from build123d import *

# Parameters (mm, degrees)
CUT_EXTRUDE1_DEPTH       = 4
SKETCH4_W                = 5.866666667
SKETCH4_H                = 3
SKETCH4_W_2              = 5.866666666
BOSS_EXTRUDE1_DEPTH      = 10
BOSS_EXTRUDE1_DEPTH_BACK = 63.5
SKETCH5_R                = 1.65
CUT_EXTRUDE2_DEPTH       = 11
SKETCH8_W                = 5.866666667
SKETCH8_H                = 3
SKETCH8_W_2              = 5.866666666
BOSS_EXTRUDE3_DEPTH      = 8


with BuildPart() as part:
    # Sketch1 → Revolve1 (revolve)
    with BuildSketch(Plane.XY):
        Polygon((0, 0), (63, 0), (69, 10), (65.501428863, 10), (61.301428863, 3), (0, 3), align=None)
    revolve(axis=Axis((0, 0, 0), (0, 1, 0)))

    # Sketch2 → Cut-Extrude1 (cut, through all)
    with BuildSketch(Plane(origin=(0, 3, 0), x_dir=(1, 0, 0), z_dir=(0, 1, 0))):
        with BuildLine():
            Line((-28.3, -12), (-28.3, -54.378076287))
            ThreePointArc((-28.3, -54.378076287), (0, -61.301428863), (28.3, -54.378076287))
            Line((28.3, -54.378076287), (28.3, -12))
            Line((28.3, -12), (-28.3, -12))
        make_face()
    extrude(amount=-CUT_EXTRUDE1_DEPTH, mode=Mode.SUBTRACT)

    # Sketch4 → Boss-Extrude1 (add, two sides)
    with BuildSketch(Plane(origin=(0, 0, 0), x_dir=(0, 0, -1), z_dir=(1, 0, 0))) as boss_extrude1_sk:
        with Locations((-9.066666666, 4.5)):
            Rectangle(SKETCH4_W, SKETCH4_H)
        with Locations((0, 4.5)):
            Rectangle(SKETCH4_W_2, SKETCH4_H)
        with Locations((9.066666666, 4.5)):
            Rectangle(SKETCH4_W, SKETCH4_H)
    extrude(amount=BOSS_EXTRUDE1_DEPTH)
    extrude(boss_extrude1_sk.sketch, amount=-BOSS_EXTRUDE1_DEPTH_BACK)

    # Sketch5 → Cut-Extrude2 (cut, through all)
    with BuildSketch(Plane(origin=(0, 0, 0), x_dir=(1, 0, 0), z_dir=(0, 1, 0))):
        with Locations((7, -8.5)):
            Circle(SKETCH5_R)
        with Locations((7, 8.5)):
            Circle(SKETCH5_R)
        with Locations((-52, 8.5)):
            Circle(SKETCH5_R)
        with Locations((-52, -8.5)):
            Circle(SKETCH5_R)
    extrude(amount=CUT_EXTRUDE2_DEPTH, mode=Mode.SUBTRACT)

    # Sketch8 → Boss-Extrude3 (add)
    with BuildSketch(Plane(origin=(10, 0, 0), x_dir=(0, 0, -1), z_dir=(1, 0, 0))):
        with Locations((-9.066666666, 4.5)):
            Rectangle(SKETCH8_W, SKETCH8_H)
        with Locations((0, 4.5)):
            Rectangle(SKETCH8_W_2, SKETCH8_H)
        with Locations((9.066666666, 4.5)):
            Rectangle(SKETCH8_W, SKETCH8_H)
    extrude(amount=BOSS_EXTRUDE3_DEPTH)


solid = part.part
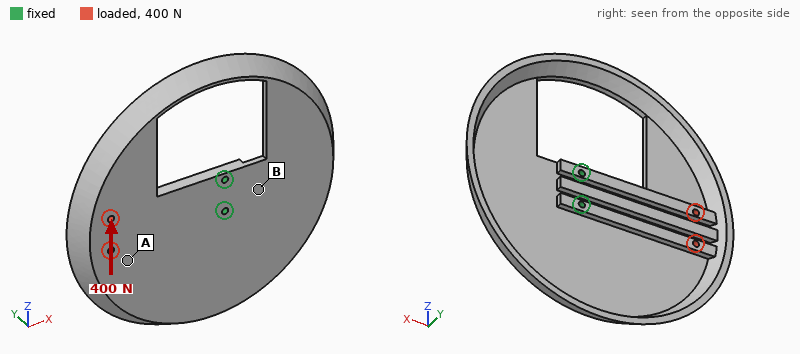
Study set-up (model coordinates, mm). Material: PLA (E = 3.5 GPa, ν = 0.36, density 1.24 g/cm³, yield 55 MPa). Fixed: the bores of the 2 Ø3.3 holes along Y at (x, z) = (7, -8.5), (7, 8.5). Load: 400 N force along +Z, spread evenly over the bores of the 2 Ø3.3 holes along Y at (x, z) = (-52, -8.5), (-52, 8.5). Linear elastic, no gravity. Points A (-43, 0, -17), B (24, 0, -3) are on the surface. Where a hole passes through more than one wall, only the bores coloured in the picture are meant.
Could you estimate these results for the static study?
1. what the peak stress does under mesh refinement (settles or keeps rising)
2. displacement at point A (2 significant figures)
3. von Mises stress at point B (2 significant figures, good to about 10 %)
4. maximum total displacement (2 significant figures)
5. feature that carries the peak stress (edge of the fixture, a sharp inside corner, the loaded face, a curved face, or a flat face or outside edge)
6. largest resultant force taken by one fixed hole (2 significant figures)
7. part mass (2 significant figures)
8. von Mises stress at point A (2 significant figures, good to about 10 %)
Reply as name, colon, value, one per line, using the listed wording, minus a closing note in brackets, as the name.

what the peak stress does under mesh refinement: keeps rising
displacement at point A: 0.52 mm
von Mises stress at point B: 8.5 MPa
maximum total displacement: 1.1 mm
feature that carries the peak stress: edge of the fixture
largest resultant force taken by one fixed hole: 1.2 kN
part mass: 55 g
von Mises stress at point A: 2.8 MPa
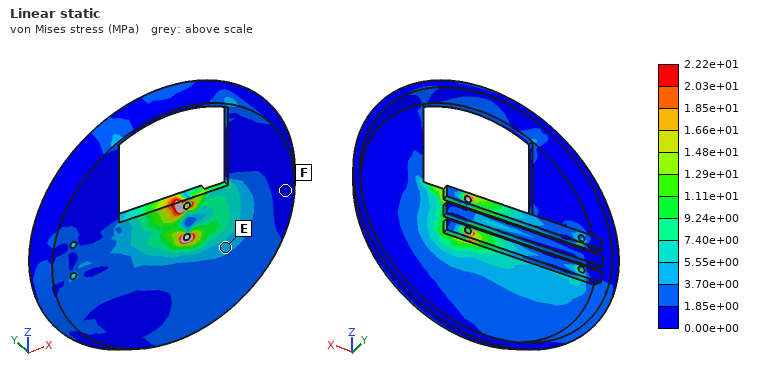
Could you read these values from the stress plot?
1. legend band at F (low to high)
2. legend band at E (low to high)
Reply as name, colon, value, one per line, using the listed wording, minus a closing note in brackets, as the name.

legend band at F: 0.00e+00 to 1.85e+00 MPa
legend band at E: 3.70e+00 to 5.55e+00 MPa
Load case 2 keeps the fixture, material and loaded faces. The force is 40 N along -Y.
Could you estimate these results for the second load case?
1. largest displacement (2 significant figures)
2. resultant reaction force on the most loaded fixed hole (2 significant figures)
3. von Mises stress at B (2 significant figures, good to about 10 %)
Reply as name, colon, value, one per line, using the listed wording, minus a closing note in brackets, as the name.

largest displacement: 2.0 mm
resultant reaction force on the most loaded fixed hole: 31 N
von Mises stress at B: 3.2 MPa
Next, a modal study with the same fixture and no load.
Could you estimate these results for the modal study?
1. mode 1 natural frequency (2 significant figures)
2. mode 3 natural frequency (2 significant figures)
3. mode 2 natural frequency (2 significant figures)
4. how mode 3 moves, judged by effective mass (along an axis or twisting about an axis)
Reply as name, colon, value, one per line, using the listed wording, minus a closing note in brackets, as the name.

mode 1 natural frequency: 180 Hz
mode 3 natural frequency: 290 Hz
mode 2 natural frequency: 200 Hz
how mode 3 moves, judged by effective mass: along Y
